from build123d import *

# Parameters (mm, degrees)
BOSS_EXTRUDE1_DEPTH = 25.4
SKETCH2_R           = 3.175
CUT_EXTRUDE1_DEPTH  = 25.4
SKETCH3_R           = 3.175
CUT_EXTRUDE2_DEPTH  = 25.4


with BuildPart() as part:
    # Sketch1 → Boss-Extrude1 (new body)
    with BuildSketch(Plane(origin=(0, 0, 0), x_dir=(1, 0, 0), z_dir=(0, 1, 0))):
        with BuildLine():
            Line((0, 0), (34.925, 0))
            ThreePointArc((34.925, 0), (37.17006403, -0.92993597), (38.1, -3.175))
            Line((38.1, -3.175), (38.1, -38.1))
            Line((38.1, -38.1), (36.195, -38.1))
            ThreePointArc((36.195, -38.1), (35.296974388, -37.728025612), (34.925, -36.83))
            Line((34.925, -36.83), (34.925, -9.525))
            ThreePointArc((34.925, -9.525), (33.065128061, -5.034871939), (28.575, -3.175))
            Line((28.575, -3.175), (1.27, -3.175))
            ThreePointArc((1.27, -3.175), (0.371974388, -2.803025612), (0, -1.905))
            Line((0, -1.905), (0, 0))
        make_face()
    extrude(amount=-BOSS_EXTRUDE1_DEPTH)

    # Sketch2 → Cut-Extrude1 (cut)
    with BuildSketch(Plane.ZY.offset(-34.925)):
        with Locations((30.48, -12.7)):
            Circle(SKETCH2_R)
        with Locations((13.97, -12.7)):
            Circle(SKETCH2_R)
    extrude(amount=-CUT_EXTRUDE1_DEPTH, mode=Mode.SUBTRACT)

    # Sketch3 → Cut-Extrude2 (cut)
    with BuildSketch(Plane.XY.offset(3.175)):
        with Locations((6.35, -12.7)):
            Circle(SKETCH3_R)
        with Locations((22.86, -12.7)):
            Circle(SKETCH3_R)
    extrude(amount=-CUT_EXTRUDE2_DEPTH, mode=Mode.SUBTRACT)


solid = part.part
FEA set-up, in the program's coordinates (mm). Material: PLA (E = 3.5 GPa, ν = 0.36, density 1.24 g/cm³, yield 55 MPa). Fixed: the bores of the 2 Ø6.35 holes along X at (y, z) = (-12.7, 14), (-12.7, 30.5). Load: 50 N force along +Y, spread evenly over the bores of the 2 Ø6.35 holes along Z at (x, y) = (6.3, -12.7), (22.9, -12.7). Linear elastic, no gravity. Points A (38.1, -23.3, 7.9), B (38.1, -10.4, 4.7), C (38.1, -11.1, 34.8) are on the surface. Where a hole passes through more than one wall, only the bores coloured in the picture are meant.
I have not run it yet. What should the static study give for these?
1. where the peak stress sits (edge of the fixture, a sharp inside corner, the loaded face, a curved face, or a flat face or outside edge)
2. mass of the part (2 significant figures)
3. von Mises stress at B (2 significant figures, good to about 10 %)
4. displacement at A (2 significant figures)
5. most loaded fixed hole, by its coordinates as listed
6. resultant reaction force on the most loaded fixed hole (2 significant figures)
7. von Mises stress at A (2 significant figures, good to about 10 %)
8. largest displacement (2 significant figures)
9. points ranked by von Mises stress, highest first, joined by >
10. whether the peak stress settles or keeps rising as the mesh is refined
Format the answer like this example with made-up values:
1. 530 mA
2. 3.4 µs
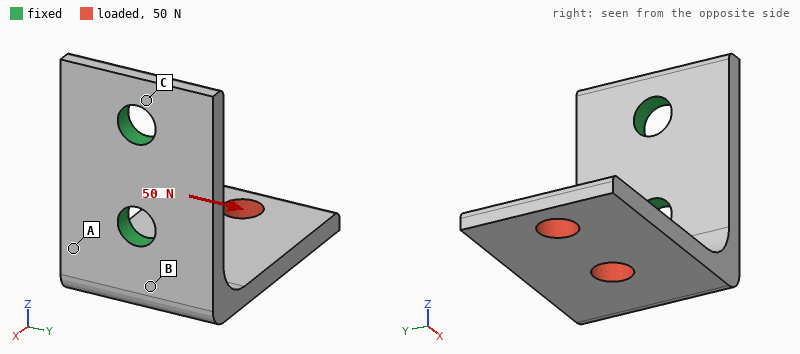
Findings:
1. edge of the fixture
2. 7.0 g
3. 9.0 MPa
4. 0.13 mm
5. (-12.7, 14)
6. 68 N
7. 5.1 MPa
8. 0.68 mm
9. B > A > C
10. keeps rising
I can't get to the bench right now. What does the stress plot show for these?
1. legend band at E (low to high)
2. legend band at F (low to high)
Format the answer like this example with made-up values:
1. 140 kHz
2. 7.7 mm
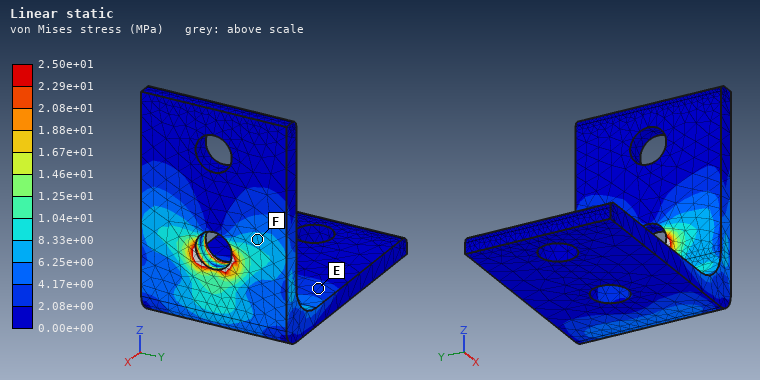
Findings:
1. 2.08e+00 to 4.17e+00 MPa
2. 6.25e+00 to 8.33e+00 MPa
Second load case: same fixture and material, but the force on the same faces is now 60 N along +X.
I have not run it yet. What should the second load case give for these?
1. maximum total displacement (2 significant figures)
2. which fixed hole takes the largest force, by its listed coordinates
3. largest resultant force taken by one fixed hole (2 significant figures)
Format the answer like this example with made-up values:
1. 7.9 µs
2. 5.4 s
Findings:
1. 0.48 mm
2. (-12.7, 14)
3. 67 N
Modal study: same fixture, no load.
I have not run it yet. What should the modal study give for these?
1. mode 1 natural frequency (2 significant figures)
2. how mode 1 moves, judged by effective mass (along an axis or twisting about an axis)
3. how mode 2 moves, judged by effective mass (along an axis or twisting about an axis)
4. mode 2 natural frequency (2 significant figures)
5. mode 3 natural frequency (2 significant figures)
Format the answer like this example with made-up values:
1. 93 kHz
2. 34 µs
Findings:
1. 560 Hz
2. along Z
3. along Y
4. 960 Hz
5. 2000 Hz
